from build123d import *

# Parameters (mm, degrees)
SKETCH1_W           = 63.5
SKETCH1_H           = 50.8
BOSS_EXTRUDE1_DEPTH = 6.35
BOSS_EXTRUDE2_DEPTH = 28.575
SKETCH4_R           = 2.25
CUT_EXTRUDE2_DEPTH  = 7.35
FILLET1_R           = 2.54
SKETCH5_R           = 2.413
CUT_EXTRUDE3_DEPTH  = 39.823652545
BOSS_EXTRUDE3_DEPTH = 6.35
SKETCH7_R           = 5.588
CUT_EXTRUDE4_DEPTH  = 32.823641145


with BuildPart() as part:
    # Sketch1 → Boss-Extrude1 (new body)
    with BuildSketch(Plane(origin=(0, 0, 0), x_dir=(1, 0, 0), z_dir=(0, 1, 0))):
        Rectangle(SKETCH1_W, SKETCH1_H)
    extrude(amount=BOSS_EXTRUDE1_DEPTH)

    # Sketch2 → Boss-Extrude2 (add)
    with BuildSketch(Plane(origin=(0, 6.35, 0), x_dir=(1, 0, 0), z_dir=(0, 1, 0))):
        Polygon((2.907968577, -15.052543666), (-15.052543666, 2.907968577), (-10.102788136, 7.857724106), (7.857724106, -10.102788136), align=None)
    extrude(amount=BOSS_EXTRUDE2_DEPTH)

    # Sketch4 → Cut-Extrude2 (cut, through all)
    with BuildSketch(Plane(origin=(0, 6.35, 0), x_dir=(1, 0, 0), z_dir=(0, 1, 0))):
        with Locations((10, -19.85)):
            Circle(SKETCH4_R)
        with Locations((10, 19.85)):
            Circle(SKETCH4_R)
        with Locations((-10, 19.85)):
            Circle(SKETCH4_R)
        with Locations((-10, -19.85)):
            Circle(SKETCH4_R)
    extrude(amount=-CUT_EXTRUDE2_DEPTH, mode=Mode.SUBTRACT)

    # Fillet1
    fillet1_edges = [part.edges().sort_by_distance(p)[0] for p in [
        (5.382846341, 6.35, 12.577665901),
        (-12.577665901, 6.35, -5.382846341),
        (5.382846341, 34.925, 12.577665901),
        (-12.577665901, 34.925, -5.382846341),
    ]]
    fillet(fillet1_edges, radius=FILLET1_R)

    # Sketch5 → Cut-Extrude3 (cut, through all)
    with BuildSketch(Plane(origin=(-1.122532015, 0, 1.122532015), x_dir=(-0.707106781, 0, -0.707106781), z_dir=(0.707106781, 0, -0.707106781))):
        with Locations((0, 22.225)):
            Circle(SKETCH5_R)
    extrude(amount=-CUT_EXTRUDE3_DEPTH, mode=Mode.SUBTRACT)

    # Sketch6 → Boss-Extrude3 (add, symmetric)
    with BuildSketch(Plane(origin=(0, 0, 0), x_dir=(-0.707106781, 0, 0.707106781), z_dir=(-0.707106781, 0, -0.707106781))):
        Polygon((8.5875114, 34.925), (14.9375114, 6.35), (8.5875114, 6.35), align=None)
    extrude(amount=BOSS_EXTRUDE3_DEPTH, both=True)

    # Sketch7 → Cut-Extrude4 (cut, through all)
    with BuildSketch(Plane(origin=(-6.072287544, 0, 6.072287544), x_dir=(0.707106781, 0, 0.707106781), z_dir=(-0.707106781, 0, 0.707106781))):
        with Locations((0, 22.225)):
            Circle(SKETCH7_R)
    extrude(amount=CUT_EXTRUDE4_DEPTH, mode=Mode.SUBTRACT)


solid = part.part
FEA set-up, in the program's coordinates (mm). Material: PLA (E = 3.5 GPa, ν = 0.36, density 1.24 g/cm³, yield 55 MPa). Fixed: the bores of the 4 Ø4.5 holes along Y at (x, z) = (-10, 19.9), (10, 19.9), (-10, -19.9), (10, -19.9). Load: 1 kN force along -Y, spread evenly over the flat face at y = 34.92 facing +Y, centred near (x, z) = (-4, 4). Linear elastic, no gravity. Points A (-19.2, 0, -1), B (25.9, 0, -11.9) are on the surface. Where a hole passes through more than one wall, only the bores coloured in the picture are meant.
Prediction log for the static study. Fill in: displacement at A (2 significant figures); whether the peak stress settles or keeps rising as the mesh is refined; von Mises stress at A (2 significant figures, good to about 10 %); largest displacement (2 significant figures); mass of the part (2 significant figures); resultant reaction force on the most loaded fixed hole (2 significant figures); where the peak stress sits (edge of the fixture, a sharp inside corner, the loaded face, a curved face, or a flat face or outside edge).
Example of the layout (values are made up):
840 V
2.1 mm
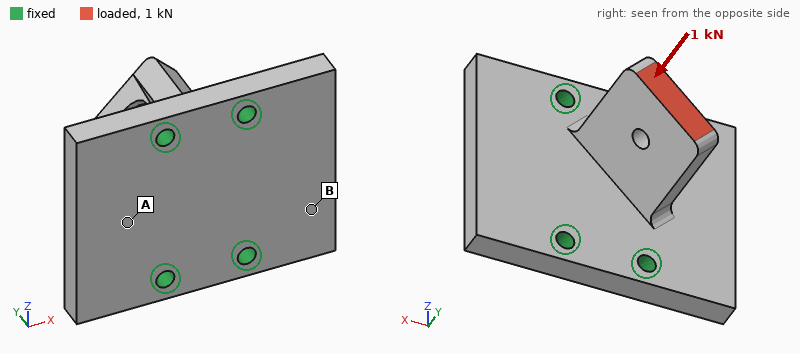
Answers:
0.083 mm
keeps rising
5.9 MPa
0.21 mm
32 g
330 N
edge of the fixture
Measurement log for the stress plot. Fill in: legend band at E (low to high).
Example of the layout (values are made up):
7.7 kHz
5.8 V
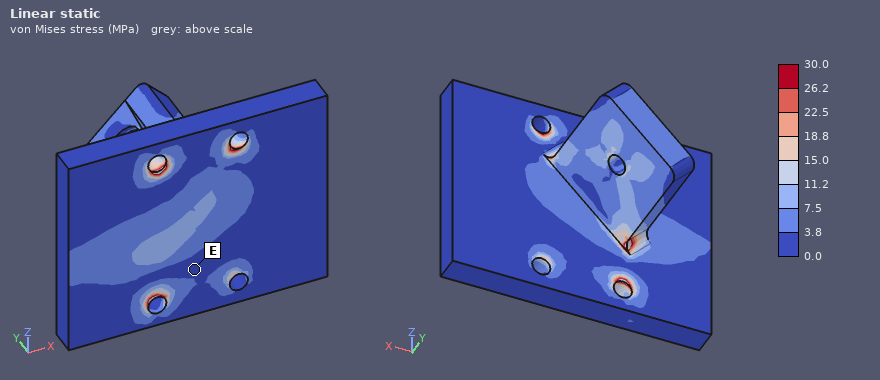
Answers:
0.0 to 3.8 MPa
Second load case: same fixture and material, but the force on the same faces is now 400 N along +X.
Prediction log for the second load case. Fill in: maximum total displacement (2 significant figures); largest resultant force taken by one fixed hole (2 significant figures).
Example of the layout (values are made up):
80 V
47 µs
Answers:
0.73 mm
460 N
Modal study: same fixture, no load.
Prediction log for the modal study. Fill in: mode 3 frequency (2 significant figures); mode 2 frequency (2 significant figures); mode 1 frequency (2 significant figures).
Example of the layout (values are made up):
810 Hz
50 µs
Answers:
3000 Hz
2900 Hz
2400 Hz
